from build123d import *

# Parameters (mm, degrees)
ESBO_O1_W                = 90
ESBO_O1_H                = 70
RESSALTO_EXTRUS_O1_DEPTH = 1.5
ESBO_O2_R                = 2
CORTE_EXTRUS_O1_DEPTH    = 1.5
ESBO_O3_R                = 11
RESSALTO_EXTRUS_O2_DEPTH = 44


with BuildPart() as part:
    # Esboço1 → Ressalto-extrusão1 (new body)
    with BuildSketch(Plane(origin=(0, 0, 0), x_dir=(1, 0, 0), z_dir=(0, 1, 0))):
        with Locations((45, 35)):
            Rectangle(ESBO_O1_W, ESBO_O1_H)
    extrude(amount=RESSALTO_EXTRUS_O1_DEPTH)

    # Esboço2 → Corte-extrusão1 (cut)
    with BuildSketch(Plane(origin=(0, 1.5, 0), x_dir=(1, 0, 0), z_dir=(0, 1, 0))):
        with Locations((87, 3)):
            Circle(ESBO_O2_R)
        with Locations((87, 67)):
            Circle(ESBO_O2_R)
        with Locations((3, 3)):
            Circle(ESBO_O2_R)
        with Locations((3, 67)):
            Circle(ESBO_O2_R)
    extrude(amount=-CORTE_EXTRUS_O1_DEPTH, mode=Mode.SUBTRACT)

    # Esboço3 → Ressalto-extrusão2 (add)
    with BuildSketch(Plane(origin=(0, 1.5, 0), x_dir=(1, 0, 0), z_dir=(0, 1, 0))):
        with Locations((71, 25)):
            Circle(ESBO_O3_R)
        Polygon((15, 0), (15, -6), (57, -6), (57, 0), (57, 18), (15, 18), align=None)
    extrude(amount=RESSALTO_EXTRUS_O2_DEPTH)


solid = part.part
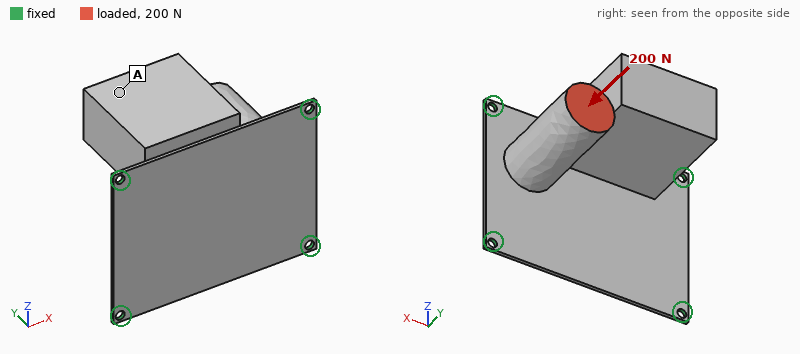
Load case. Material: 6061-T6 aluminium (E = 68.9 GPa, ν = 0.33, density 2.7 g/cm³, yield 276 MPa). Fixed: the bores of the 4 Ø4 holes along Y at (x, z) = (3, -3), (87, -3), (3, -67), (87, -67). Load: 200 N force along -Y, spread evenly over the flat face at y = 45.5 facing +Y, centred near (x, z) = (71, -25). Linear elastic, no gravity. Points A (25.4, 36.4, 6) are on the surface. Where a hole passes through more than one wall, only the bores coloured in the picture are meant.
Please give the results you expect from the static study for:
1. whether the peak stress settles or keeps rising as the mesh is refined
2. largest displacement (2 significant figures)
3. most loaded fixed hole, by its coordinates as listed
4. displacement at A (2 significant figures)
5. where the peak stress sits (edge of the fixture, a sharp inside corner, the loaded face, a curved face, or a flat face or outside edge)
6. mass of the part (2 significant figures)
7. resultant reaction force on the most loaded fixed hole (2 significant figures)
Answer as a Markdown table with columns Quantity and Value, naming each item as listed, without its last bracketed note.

| Quantity | Value |
|---|---|
| whether the peak stress settles or keeps rising as the mesh is refined | keeps rising |
| largest displacement | 0.38 mm |
| most loaded fixed hole, by its coordinates as listed | (87, -3) |
| displacement at A | 0.22 mm |
| where the peak stress sits | edge of the fixture |
| mass of the part | 190 g |
| resultant reaction force on the most loaded fixed hole | 130 N |
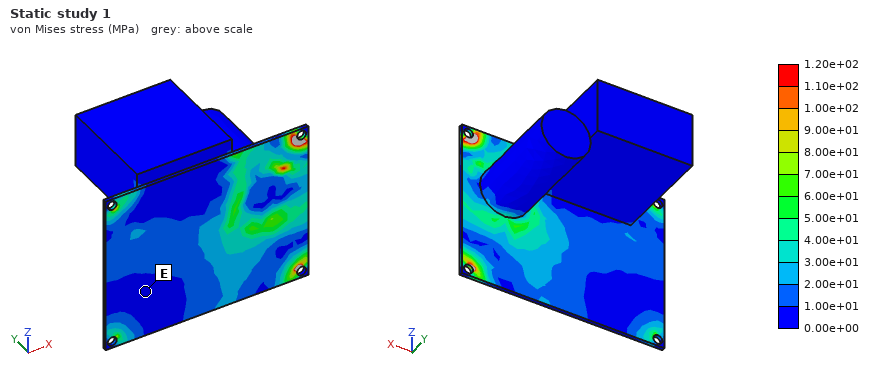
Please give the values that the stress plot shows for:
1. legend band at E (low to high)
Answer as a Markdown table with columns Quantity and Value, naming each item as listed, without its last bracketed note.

| Quantity | Value |
|---|---|
| legend band at E | 0.00e+00 to 1.00e+01 MPa |
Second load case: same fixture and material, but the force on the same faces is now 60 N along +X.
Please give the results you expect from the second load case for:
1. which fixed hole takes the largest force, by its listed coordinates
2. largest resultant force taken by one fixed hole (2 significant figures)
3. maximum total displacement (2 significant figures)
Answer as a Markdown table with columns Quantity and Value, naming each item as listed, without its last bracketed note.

| Quantity | Value |
|---|---|
| which fixed hole takes the largest force, by its listed coordinates | (3, -3) |
| largest resultant force taken by one fixed hole | 46 N |
| maximum total displacement | 0.45 mm |
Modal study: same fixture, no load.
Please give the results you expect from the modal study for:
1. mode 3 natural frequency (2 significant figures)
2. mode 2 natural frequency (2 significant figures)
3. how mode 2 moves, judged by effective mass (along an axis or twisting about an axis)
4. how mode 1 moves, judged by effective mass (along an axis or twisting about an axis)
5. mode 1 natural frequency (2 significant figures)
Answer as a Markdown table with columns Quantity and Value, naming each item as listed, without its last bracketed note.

| Quantity | Value |
|---|---|
| mode 3 natural frequency | 560 Hz |
| mode 2 natural frequency | 330 Hz |
| how mode 2 moves, judged by effective mass | along Y |
| how mode 1 moves, judged by effective mass | along Z |
| mode 1 natural frequency | 270 Hz |
